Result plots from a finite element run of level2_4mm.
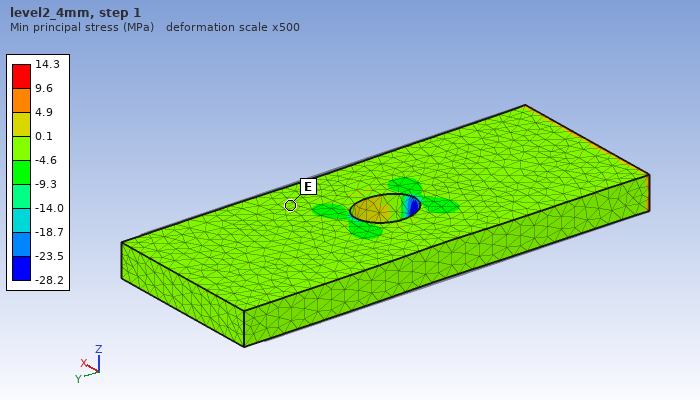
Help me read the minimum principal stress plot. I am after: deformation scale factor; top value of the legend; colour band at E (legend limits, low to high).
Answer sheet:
500
14.3 MPa
-4.6 to 0.1 MPa
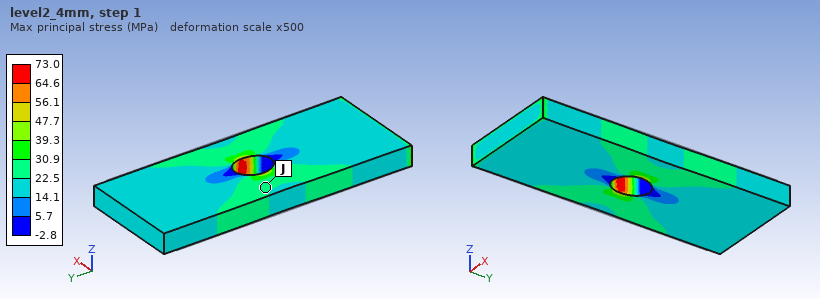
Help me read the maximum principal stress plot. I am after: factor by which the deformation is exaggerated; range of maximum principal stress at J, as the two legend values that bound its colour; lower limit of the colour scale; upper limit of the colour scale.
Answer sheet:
500
22.5 to 30.9 MPa
-2.8 MPa
73.0 MPa
